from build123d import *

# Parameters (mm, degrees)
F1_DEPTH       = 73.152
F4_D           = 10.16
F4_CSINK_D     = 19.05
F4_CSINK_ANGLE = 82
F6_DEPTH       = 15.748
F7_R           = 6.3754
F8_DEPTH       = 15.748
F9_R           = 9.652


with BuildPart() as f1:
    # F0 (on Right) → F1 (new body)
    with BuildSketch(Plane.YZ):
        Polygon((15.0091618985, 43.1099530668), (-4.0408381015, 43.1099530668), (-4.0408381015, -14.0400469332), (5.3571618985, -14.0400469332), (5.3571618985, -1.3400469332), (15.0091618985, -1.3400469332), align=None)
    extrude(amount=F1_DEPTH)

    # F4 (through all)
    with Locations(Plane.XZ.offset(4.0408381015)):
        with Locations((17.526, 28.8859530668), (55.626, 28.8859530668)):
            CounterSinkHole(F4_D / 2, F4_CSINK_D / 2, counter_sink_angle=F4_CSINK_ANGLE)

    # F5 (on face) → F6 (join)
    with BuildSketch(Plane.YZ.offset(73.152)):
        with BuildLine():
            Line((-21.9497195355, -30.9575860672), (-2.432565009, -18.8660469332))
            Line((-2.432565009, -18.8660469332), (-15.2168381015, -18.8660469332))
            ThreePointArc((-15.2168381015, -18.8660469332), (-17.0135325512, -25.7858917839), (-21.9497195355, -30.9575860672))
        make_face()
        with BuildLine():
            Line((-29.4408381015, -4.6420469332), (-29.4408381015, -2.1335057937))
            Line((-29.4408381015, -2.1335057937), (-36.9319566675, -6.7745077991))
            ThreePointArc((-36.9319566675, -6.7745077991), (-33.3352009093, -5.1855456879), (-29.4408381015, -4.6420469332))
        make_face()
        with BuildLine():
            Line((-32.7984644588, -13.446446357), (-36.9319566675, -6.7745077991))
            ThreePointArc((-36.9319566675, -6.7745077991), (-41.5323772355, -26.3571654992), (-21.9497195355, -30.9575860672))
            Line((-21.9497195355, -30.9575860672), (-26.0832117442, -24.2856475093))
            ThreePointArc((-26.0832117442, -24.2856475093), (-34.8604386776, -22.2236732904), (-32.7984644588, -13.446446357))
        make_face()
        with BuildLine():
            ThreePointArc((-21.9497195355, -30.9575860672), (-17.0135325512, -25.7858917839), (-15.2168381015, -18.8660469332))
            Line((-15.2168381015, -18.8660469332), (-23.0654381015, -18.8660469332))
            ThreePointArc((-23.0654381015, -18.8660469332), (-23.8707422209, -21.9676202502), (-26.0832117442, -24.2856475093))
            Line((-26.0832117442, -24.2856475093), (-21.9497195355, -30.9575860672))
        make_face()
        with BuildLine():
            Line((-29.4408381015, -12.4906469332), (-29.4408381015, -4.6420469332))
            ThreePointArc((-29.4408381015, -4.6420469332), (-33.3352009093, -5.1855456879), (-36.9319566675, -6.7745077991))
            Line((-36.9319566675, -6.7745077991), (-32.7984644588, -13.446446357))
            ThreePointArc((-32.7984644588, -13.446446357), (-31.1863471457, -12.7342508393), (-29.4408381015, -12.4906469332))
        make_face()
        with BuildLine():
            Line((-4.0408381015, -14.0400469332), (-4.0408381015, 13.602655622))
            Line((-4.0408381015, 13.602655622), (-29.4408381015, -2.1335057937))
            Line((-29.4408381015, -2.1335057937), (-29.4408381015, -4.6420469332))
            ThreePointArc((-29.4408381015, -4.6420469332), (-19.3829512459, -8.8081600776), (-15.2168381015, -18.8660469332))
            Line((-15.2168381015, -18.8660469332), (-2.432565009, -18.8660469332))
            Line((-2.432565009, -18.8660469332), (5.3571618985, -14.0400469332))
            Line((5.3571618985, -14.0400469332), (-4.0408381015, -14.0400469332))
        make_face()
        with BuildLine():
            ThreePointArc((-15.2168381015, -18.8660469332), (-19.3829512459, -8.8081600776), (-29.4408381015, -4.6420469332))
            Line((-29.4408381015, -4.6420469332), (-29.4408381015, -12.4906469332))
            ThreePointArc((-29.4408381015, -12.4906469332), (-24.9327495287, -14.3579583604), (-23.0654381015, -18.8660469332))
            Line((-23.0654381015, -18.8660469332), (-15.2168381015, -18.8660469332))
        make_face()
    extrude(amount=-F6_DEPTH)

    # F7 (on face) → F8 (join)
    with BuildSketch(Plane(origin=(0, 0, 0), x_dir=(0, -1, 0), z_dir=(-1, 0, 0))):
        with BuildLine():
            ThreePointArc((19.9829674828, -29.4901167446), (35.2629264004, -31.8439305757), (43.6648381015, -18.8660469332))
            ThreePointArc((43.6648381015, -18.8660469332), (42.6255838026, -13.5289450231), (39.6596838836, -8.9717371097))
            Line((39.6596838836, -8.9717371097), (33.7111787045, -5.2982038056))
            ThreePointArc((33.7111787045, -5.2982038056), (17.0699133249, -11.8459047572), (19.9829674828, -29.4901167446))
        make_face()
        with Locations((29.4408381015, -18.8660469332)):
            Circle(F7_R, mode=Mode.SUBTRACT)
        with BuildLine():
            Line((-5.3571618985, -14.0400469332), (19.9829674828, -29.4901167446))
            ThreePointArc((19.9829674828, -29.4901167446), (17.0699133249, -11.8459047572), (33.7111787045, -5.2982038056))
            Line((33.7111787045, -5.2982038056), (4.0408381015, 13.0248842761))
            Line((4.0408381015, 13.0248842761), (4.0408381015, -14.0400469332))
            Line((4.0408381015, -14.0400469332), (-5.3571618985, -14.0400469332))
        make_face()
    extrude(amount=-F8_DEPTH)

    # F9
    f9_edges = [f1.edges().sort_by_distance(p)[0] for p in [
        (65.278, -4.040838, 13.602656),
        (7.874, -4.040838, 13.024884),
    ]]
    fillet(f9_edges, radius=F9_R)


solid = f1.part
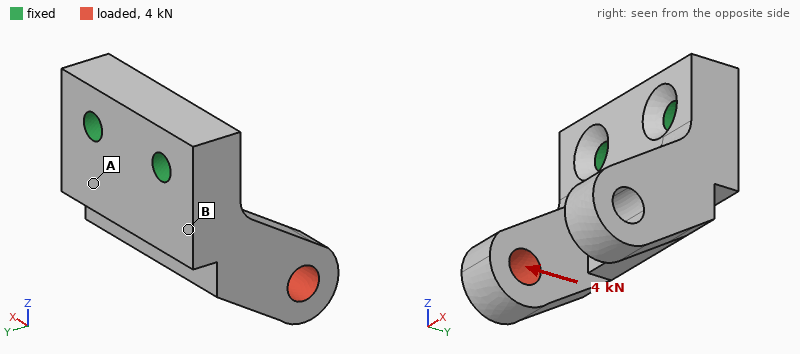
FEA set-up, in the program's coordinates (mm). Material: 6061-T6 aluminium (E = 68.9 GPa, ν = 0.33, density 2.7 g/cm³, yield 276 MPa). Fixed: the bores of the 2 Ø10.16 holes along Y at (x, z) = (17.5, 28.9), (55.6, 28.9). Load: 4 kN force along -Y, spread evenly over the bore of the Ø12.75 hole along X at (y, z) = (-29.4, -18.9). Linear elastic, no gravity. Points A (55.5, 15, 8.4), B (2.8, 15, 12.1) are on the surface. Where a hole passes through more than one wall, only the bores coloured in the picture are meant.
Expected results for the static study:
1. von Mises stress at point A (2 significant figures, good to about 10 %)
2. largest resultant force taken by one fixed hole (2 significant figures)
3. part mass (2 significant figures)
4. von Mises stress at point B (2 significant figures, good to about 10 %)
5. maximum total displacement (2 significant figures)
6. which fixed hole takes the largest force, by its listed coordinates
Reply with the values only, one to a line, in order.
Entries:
16 MPa
4.2 kN
270 g
44 MPa
0.29 mm
(17.5, 28.9)
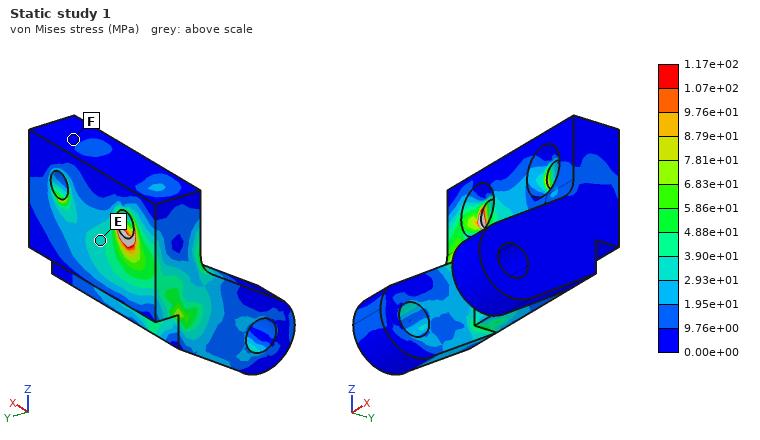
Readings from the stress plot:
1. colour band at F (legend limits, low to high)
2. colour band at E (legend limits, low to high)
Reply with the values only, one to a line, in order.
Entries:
0.00e+00 to 9.76e+00 MPa
2.93e+01 to 3.90e+01 MPa
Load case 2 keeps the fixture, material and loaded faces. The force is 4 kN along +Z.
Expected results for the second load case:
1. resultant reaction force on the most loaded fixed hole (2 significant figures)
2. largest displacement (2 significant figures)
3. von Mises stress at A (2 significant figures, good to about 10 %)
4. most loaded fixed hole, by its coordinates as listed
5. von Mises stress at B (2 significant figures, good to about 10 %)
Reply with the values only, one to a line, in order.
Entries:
4.5 kN
0.29 mm
14 MPa
(17.5, 28.9)
45 MPa
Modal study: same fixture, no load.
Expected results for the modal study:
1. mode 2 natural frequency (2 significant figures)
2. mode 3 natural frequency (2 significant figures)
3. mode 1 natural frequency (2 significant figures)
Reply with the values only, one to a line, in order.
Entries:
3200 Hz
4200 Hz
2900 Hz
